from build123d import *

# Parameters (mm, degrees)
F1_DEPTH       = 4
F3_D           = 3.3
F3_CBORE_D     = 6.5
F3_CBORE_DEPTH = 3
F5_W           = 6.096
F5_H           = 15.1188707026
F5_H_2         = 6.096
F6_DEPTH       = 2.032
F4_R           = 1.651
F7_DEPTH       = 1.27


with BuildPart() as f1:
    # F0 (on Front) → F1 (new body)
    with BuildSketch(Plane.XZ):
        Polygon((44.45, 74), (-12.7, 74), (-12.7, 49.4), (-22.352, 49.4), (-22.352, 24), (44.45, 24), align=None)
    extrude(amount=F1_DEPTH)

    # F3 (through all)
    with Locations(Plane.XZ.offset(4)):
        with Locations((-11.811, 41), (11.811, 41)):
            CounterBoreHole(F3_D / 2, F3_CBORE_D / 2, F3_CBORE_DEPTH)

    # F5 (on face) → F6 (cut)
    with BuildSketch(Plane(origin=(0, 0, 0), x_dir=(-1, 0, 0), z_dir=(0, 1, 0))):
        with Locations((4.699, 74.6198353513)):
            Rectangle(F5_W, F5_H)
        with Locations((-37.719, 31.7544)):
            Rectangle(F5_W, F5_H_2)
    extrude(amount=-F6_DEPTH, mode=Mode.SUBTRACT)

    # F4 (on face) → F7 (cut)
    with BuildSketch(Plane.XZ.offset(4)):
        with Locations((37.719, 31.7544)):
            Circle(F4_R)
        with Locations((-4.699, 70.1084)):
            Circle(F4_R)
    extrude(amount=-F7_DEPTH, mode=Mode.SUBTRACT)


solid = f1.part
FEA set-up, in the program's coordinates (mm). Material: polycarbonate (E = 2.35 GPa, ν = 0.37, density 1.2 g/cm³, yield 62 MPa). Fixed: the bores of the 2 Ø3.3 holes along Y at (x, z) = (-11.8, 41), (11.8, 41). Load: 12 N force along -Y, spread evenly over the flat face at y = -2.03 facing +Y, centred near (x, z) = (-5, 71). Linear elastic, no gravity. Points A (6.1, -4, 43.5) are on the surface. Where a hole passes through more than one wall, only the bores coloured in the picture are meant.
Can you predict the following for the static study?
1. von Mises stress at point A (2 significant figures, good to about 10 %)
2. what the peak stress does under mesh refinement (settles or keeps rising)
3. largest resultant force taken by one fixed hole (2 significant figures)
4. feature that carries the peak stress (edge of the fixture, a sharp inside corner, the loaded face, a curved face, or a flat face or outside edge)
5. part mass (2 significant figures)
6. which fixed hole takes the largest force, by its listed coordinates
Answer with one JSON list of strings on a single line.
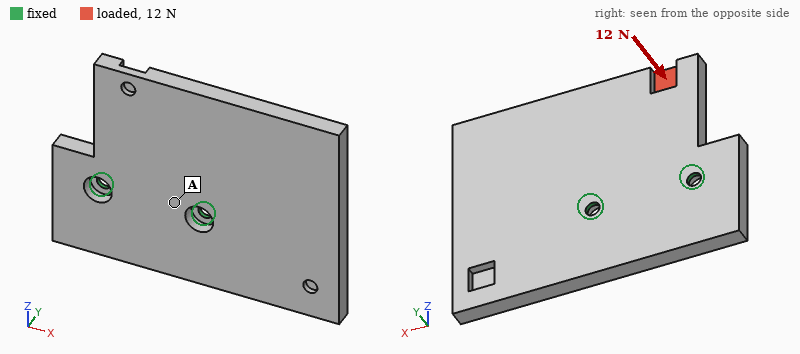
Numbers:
["3.7 MPa", "keeps rising", "12 N", "edge of the fixture", "14 g", "(-11.8, 41)"]
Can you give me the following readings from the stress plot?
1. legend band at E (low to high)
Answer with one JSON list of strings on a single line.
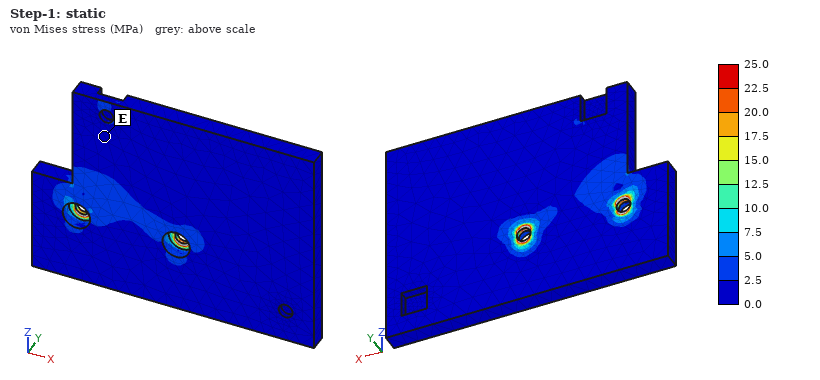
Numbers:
["0.0 to 2.5 MPa"]
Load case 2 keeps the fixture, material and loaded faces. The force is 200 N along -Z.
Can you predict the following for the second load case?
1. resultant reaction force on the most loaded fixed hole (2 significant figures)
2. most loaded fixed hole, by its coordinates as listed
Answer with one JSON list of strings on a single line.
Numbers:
["140 N", "(-11.8, 41)"]
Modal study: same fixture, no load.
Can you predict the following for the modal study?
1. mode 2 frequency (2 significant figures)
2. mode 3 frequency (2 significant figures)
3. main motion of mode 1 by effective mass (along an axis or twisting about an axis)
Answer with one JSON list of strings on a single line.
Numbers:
["600 Hz", "1200 Hz", "along Y"]
